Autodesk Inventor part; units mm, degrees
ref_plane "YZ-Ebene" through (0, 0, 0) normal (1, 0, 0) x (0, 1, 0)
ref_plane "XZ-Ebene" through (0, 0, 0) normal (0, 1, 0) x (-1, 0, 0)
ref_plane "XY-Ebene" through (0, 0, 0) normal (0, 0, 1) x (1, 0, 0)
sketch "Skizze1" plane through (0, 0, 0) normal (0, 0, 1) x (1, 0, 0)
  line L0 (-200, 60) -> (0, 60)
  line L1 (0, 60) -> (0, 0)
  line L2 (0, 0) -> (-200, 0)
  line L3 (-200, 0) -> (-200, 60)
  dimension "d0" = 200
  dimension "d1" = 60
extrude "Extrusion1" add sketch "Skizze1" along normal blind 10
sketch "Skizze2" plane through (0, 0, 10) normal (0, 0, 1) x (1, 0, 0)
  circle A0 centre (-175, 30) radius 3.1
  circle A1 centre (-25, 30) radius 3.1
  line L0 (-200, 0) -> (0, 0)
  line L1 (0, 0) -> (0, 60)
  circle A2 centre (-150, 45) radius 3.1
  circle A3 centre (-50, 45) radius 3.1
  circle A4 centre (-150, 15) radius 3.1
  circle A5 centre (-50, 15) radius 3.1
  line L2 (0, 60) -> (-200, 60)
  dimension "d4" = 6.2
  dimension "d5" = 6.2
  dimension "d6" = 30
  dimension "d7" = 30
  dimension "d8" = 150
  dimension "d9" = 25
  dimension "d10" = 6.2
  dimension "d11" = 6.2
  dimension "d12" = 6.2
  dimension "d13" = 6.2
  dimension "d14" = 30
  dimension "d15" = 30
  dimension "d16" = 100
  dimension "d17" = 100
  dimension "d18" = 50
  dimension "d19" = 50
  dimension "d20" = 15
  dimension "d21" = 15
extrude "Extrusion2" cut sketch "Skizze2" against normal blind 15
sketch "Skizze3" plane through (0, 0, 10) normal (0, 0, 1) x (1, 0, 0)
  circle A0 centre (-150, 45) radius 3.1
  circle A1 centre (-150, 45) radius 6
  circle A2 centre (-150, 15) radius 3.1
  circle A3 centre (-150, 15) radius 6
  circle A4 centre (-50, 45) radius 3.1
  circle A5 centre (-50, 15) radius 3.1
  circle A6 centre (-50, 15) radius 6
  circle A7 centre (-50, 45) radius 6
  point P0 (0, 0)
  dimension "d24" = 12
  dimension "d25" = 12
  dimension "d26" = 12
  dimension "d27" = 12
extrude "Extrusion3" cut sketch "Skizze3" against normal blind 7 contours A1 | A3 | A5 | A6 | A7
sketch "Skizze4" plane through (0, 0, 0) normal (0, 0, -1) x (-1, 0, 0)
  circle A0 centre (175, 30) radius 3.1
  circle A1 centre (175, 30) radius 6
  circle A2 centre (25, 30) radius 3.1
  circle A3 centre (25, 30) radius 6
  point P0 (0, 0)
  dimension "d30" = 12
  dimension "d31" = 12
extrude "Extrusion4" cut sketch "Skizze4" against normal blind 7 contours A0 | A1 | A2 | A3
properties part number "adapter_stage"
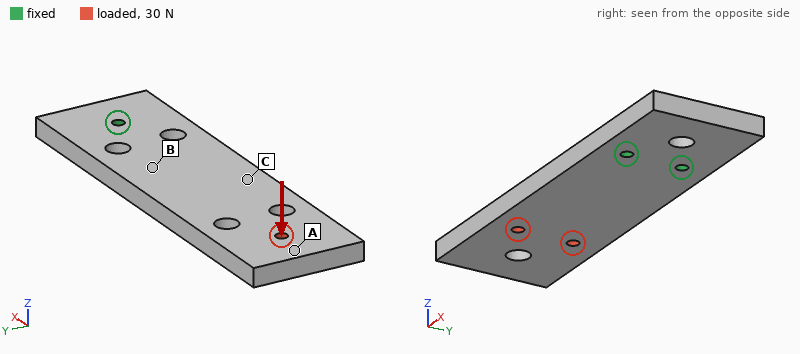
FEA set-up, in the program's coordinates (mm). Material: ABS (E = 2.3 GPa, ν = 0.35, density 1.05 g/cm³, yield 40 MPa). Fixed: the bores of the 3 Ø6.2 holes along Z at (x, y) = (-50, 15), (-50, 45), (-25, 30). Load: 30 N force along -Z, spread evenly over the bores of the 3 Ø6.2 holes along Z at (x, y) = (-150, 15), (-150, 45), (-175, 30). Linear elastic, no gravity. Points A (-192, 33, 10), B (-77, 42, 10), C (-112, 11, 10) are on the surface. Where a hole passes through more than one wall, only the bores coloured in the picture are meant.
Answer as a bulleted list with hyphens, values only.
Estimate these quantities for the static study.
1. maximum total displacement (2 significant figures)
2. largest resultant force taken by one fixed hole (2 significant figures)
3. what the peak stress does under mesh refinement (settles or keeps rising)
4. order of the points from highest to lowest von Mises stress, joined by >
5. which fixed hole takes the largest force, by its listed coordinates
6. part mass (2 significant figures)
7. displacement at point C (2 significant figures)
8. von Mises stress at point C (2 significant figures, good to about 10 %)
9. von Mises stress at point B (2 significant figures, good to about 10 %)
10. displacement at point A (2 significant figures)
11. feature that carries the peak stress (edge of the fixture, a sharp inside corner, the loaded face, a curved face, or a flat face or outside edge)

- 2.2 mm
- 130 N
- keeps rising
- B > C > A
- (-25, 30)
- 120 g
- 0.63 mm
- 1.4 MPa
- 2.3 MPa
- 2.1 mm
- edge of the fixture
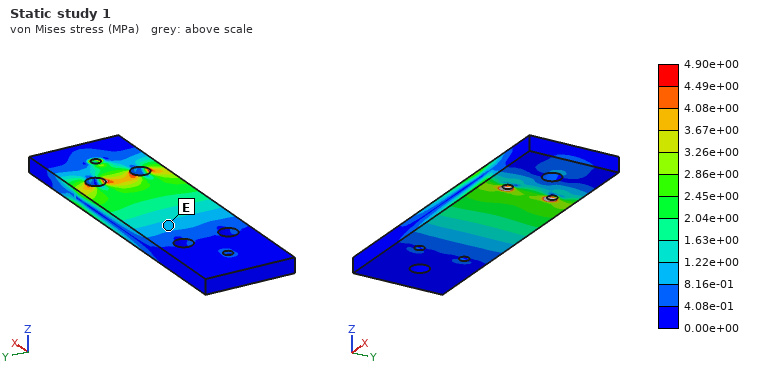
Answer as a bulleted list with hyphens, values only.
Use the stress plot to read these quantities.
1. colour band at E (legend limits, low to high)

- 8.16e-01 to 1.22e+00 MPa
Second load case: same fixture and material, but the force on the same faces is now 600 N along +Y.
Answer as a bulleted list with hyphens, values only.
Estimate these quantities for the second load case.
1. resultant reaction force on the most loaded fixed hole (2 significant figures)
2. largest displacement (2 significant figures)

- 1.6 kN
- 2.0 mm
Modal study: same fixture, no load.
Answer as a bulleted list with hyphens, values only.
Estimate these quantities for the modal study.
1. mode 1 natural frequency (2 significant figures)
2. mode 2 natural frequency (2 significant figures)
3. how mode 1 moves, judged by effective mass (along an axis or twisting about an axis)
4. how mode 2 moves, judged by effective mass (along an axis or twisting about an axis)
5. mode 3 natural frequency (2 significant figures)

- 96 Hz
- 430 Hz
- along Z
- along Y
- 490 Hz
